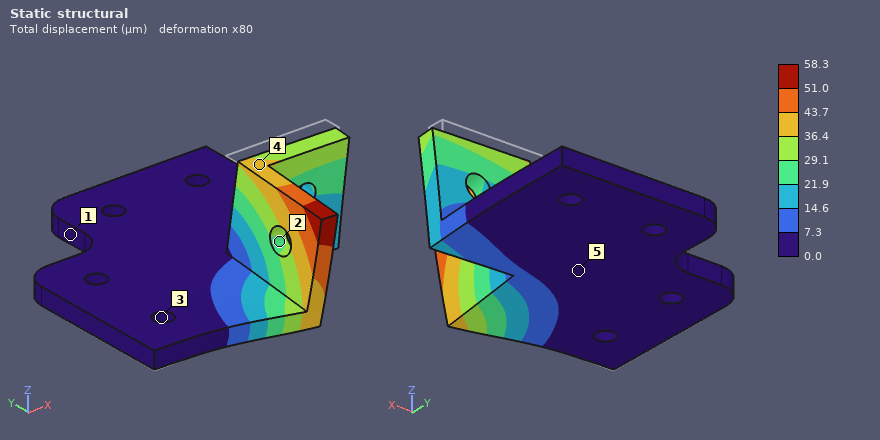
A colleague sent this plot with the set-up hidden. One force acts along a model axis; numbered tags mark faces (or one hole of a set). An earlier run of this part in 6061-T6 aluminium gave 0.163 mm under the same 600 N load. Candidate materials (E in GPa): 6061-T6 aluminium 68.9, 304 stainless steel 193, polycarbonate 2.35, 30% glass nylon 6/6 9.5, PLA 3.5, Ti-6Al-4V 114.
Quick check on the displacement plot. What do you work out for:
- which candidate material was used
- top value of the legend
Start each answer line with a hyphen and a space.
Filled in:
- 304 stainless steel
- 58.3 µm
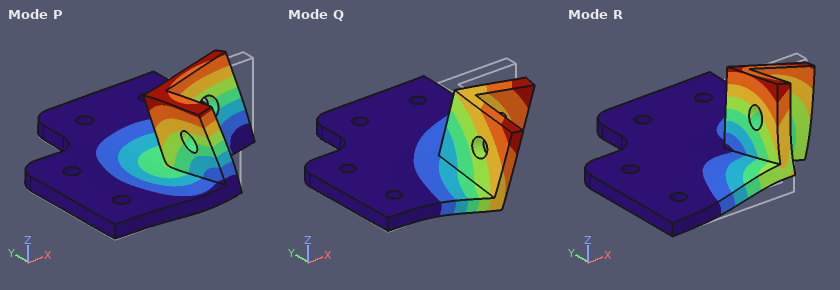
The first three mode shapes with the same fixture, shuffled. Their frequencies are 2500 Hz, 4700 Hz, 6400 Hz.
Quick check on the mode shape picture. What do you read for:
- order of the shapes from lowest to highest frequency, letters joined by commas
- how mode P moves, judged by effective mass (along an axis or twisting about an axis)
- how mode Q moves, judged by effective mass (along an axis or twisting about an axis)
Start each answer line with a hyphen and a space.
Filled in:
- Q, R, P
- along Z
- along Z
